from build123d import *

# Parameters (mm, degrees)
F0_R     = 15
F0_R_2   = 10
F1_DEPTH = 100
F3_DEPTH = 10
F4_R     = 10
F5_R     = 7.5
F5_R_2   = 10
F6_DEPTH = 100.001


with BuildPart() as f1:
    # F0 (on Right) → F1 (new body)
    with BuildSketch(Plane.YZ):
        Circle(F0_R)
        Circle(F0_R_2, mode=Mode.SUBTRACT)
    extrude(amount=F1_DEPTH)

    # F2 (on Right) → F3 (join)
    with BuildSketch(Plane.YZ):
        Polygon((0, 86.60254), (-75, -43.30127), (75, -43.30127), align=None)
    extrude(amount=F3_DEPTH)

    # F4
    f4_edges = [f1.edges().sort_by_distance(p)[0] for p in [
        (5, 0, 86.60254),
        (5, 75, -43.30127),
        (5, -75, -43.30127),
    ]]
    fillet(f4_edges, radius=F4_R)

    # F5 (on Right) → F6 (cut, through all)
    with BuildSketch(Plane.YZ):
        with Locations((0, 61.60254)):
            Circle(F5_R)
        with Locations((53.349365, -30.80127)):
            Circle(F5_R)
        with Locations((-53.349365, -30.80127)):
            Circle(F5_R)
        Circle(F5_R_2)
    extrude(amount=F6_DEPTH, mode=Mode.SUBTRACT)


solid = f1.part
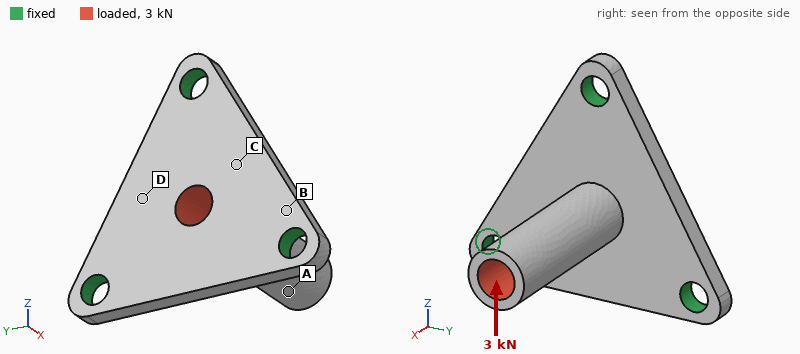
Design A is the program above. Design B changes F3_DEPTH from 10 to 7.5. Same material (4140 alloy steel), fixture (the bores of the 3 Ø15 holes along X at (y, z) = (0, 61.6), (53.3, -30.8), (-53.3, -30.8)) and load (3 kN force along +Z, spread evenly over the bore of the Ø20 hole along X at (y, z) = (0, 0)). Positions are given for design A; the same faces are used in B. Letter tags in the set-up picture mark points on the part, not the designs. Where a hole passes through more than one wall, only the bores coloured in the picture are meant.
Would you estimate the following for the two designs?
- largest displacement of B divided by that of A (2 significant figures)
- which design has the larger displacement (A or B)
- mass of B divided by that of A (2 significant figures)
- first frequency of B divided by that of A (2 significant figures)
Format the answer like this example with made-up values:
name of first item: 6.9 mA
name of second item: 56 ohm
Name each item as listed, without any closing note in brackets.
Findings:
largest displacement of B divided by that of A: 1.7
which design has the larger displacement: B
mass of B divided by that of A: 0.83
first frequency of B divided by that of A: 0.76
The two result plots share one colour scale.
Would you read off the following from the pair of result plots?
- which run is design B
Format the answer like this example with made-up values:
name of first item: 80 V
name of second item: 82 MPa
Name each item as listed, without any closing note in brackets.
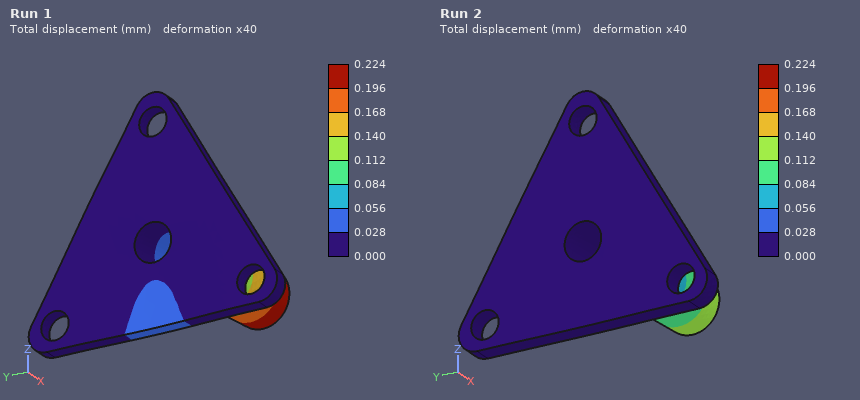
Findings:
which run is design B: Run 1
